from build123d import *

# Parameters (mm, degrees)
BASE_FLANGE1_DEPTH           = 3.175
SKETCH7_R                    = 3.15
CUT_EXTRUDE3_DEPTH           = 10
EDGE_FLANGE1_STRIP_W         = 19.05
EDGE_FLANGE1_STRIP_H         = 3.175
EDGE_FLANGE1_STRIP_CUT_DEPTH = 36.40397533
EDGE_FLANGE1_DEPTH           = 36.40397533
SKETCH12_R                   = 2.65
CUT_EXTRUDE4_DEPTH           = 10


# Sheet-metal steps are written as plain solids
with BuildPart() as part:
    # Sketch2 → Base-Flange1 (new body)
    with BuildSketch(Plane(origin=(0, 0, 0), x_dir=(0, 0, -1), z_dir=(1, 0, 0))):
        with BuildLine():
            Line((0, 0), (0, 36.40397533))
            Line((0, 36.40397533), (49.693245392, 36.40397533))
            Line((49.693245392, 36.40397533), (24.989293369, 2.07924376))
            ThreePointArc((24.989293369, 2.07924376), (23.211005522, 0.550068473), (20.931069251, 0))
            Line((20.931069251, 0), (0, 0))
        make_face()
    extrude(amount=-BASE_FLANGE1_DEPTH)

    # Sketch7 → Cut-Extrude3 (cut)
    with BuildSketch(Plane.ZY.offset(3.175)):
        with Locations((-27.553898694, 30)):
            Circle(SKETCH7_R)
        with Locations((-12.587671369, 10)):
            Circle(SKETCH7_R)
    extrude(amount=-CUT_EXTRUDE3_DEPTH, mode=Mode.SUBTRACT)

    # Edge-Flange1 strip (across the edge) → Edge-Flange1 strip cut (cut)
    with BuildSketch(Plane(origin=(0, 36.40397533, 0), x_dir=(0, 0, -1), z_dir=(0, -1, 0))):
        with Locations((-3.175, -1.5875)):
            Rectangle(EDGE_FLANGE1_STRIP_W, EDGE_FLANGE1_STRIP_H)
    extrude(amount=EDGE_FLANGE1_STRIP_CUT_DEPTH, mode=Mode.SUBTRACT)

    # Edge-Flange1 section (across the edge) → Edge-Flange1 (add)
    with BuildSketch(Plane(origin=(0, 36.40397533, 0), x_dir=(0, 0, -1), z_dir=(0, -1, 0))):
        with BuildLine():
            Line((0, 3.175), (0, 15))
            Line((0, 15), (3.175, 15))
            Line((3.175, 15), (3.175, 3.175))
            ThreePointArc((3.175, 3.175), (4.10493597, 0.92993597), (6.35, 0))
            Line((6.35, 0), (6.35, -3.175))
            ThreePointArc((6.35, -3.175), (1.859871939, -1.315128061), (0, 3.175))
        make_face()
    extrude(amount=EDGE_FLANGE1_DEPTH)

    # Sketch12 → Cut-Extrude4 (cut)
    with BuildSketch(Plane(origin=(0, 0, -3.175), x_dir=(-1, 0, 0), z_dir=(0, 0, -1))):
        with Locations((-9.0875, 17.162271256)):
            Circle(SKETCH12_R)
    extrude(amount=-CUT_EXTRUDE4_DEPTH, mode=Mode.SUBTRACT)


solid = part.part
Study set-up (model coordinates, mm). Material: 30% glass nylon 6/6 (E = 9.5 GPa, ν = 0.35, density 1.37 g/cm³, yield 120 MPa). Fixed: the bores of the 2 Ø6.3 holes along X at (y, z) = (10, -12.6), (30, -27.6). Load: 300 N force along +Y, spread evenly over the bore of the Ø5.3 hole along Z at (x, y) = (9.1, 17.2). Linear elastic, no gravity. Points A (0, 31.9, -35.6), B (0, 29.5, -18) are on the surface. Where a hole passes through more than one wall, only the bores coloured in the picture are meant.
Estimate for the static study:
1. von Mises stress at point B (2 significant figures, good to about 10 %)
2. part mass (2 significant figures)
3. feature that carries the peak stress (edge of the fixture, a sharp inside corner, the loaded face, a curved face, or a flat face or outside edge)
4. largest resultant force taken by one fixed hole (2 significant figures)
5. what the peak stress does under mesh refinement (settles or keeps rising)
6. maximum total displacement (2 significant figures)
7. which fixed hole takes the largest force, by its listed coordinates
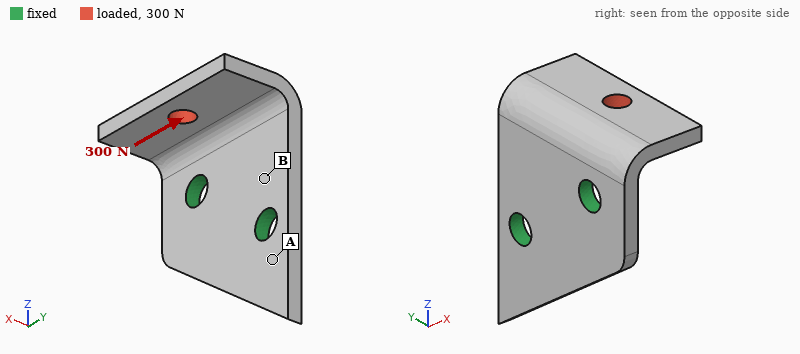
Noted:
19 MPa
7.5 g
edge of the fixture
320 N
keeps rising
0.55 mm
(10, -12.6)
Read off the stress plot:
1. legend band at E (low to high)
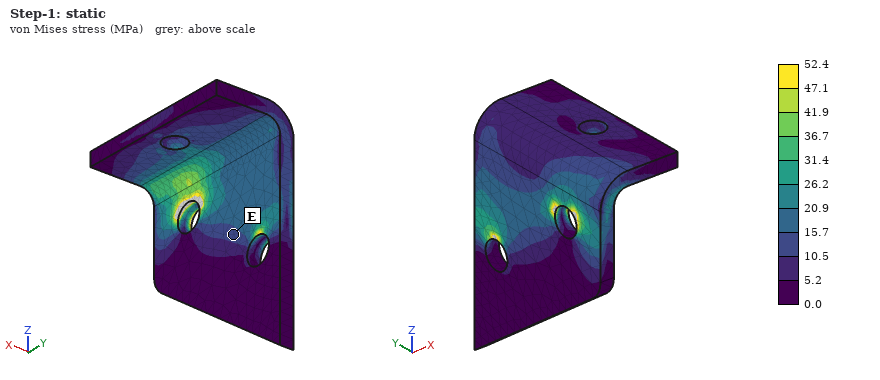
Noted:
10.5 to 15.7 MPa
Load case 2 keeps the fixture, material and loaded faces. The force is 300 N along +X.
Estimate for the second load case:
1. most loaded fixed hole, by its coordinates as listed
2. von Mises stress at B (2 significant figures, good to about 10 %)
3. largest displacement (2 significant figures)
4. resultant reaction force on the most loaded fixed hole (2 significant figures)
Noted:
(10, -12.6)
20 MPa
0.61 mm
290 N
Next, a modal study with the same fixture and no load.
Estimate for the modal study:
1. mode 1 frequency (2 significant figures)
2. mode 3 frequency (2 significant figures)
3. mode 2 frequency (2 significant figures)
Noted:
2100 Hz
5300 Hz
3300 Hz
